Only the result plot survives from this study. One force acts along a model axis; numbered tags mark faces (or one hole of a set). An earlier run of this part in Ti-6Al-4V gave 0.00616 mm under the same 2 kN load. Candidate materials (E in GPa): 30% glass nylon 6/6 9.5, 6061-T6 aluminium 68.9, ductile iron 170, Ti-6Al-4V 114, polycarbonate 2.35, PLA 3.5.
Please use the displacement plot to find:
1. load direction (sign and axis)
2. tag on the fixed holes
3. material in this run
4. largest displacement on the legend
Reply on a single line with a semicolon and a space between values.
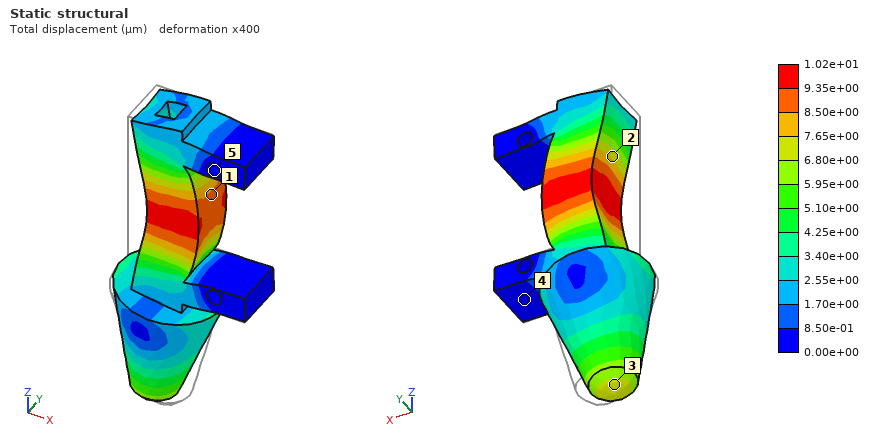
+X; 5; 6061-T6 aluminium; 1.02e+01 µm
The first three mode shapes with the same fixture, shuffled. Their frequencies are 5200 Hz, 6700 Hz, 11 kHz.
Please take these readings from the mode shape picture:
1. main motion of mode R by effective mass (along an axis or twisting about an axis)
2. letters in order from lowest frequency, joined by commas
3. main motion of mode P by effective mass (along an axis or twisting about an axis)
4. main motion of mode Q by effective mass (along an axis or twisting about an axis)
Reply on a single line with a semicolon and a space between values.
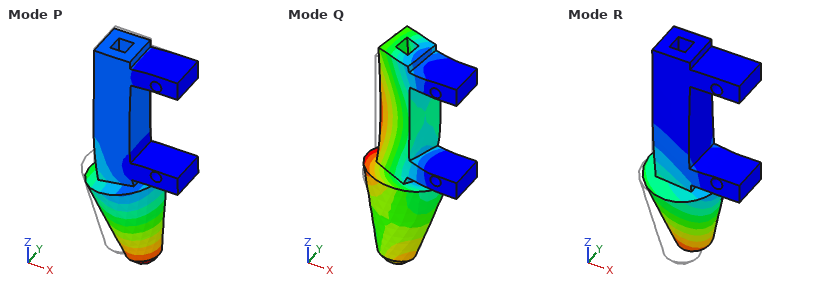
along Y; R, P, Q; along X; along Y
